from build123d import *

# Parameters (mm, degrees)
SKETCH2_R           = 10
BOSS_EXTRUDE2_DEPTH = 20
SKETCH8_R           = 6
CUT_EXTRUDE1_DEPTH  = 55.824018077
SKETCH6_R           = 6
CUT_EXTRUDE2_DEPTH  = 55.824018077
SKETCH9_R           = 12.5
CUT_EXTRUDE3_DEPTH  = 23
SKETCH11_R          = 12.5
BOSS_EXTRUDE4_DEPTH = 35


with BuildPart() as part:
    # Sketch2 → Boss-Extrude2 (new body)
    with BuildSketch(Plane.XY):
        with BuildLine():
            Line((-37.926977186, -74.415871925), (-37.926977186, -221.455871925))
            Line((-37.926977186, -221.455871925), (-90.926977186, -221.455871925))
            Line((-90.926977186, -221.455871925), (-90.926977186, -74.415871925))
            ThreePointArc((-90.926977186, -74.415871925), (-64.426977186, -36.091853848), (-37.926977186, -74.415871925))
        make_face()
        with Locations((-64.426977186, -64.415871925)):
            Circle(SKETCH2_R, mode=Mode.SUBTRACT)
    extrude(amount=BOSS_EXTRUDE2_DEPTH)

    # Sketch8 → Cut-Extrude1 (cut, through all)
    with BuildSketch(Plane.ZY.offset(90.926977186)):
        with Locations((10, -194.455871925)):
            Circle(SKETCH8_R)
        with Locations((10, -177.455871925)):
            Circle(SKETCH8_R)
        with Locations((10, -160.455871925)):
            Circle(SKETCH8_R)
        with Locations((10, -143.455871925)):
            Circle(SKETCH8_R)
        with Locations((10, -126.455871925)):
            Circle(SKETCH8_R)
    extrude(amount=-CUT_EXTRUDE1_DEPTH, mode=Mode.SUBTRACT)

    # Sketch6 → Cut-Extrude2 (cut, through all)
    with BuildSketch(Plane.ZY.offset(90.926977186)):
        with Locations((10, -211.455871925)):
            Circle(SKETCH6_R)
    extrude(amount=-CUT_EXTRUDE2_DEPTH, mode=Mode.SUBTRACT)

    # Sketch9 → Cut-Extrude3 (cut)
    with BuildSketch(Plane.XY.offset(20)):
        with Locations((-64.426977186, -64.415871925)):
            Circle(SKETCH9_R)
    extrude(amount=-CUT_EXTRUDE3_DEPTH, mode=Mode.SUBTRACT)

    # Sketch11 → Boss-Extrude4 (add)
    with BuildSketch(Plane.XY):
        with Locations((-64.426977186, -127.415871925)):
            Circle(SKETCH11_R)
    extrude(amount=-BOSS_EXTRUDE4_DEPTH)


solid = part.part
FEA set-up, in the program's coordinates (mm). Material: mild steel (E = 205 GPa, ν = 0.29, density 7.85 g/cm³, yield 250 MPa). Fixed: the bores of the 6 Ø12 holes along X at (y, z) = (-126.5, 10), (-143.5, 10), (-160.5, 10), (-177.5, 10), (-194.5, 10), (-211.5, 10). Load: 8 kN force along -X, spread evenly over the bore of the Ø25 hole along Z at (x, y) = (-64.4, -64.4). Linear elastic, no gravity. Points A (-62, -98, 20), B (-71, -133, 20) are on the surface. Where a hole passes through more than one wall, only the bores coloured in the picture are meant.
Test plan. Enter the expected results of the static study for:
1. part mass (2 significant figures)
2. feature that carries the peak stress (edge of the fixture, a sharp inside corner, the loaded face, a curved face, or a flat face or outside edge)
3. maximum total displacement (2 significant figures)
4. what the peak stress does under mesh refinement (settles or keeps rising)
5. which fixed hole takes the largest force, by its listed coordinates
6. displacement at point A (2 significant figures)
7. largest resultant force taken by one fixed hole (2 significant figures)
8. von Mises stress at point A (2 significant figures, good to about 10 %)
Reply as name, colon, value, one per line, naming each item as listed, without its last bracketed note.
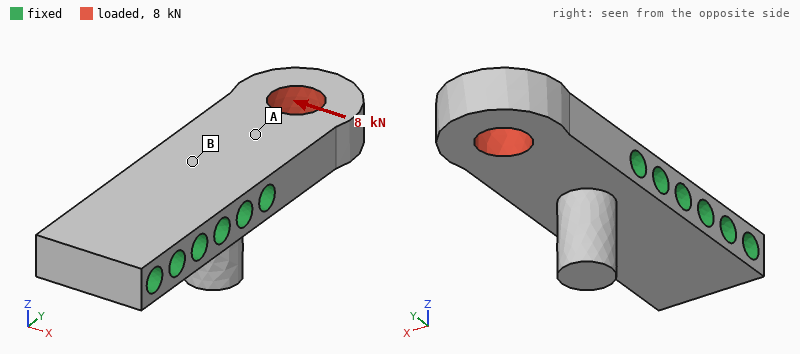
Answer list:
part mass: 1.3 kg
feature that carries the peak stress: edge of the fixture
maximum total displacement: 29 µm
what the peak stress does under mesh refinement: keeps rising
which fixed hole takes the largest force, by its listed coordinates: (-126.5, 10)
displacement at point A: 4.7 µm
largest resultant force taken by one fixed hole: 8.2 kN
von Mises stress at point A: 23 MPa
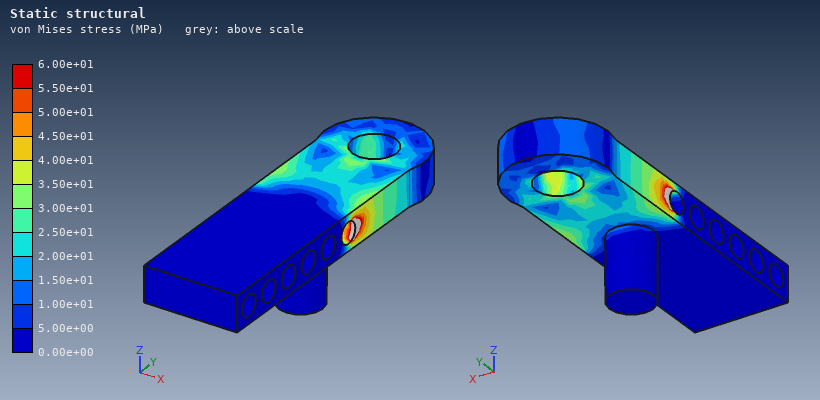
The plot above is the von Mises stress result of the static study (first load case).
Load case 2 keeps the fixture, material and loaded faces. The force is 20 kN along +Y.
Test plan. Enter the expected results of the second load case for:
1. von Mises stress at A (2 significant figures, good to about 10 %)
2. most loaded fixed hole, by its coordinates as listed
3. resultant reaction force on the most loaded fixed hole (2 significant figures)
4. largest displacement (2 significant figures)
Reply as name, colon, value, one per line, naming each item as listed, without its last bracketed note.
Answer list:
von Mises stress at A: 16 MPa
most loaded fixed hole, by its coordinates as listed: (-126.5, 10)
resultant reaction force on the most loaded fixed hole: 19 kN
largest displacement: 9.9 µm
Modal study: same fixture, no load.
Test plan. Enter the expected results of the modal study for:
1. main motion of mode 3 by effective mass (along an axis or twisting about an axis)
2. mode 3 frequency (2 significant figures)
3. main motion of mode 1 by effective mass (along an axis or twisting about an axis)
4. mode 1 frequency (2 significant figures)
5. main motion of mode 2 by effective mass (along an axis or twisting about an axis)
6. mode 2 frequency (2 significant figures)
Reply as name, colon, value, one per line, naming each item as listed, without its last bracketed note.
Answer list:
main motion of mode 3 by effective mass: twisting about Y
mode 3 frequency: 6400 Hz
main motion of mode 1 by effective mass: along Z
mode 1 frequency: 2400 Hz
main motion of mode 2 by effective mass: along X
mode 2 frequency: 5100 Hz
